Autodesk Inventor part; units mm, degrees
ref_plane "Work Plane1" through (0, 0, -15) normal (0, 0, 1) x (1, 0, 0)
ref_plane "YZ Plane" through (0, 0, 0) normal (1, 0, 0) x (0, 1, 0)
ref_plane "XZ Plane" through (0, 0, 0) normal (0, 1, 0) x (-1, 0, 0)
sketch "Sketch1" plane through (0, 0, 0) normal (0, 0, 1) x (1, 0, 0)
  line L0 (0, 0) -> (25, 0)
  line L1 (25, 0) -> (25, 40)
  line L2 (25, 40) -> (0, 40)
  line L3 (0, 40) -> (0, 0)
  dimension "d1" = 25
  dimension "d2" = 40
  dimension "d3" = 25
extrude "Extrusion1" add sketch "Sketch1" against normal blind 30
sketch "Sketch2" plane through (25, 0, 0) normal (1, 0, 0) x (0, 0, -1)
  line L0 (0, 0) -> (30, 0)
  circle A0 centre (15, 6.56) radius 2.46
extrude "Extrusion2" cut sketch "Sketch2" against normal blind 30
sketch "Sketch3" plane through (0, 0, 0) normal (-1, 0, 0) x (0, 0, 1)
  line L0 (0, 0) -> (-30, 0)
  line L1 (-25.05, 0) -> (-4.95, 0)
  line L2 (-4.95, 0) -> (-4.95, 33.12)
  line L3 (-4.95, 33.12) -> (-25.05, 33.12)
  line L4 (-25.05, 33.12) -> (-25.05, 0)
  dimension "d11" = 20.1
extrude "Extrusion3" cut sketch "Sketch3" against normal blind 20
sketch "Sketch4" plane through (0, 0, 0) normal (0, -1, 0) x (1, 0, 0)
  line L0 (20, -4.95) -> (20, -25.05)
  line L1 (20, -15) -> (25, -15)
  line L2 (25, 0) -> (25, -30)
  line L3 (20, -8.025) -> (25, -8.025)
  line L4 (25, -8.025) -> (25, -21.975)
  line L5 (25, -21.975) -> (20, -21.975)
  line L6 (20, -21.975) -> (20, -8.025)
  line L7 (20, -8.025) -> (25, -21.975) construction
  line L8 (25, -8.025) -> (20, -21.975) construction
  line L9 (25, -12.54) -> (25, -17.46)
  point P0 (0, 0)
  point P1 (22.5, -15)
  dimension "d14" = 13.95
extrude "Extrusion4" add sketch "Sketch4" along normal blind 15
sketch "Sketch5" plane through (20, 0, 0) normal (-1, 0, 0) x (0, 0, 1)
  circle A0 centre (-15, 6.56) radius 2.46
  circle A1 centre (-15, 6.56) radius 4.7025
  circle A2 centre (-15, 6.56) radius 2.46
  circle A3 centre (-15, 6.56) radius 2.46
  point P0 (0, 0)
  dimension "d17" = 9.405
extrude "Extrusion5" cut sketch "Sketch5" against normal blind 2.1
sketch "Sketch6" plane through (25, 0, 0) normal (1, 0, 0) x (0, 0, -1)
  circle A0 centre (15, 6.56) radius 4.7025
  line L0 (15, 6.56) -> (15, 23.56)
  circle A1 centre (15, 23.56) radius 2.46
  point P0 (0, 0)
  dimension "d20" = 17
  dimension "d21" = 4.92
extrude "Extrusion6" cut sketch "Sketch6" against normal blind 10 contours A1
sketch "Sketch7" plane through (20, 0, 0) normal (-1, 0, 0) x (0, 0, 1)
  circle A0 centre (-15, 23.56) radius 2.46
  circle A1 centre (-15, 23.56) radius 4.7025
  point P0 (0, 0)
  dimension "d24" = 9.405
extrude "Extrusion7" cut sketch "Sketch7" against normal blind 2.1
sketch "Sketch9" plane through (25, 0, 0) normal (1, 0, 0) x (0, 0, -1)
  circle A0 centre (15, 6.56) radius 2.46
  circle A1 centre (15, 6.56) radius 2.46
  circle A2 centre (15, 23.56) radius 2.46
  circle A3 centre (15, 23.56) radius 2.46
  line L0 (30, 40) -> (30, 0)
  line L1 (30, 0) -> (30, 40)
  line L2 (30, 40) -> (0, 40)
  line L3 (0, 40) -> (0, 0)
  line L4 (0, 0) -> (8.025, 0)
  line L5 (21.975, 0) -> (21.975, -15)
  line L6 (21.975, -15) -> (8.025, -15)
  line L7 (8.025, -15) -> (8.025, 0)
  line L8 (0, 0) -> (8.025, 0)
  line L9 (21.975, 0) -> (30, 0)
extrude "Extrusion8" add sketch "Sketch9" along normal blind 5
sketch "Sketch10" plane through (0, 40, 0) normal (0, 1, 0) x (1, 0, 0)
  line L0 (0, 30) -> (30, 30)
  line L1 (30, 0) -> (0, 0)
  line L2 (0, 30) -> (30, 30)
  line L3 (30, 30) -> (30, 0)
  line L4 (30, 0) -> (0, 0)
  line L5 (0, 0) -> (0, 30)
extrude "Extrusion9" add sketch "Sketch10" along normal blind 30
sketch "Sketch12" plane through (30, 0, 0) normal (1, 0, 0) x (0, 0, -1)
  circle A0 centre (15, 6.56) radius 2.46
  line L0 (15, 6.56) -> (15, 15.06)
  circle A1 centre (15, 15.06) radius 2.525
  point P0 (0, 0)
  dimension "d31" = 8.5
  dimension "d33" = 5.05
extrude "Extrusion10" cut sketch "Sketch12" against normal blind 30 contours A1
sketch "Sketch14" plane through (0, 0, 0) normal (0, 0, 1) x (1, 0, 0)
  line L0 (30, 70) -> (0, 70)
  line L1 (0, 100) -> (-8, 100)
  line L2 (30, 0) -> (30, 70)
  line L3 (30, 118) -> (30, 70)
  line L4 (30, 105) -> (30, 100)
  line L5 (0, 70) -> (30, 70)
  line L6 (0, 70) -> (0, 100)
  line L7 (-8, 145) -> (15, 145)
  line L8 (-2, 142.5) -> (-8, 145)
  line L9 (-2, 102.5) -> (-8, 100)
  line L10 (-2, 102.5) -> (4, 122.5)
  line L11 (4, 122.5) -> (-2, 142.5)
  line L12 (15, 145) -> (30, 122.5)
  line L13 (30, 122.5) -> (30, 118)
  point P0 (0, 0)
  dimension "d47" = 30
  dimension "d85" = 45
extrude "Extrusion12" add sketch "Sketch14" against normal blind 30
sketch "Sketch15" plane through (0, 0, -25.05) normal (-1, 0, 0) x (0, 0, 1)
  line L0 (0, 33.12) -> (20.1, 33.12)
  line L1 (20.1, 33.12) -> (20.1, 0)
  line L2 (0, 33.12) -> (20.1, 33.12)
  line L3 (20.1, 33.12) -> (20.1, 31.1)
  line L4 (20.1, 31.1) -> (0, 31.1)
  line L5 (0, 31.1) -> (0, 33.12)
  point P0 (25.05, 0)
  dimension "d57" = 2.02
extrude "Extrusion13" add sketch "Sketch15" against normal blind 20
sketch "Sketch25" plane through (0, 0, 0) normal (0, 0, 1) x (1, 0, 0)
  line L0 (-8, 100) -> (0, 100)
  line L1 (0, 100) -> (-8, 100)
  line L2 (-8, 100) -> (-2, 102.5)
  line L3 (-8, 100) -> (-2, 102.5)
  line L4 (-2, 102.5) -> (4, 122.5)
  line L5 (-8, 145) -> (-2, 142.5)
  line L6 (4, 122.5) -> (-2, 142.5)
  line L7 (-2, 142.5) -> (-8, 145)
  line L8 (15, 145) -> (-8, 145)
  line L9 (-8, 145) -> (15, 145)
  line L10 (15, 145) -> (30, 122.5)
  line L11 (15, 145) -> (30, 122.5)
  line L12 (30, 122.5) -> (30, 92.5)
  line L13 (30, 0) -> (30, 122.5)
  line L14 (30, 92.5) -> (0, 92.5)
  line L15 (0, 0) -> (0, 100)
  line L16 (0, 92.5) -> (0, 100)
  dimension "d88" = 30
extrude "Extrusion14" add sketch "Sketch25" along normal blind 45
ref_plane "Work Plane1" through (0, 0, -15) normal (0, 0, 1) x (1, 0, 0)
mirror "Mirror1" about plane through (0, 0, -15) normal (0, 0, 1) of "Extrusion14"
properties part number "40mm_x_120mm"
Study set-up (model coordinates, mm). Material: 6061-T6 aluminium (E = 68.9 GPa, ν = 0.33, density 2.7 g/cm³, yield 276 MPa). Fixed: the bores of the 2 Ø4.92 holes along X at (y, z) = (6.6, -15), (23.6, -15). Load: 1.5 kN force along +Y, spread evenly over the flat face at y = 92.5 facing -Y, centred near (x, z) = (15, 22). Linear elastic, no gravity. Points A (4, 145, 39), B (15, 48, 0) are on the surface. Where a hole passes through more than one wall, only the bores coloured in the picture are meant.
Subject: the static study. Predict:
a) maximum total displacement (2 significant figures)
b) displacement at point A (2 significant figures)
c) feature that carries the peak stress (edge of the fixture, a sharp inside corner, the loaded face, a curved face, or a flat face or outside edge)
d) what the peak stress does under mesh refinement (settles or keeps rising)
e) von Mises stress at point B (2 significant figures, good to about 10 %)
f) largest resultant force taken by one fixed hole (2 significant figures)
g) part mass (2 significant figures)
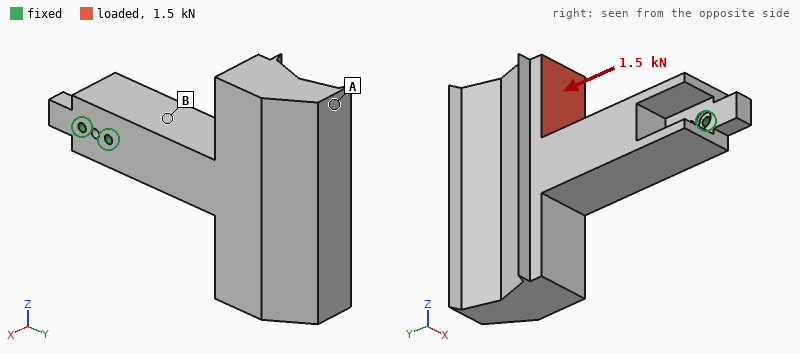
0.22 mm
0.21 mm
edge of the fixture
keeps rising
15 MPa
2.7 kN
650 g
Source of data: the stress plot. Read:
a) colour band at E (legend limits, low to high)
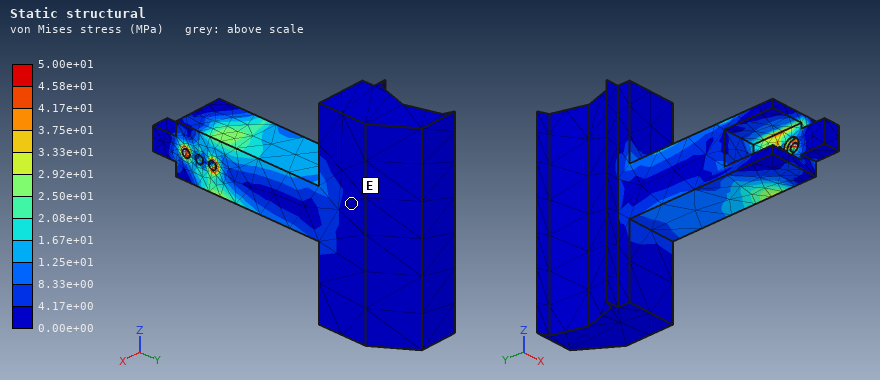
0.00e+00 to 4.17e+00 MPa
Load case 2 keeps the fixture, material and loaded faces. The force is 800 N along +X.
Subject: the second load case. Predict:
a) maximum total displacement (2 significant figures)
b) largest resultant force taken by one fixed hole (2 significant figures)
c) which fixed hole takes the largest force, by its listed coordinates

0.32 mm
3.0 kN
(23.6, -15)
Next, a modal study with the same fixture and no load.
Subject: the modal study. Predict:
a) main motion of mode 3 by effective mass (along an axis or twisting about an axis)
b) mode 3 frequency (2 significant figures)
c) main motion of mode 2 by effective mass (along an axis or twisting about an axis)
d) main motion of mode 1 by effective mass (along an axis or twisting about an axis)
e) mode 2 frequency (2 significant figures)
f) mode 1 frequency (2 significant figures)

twisting about Y
780 Hz
along Z
along X
500 Hz
460 Hz
